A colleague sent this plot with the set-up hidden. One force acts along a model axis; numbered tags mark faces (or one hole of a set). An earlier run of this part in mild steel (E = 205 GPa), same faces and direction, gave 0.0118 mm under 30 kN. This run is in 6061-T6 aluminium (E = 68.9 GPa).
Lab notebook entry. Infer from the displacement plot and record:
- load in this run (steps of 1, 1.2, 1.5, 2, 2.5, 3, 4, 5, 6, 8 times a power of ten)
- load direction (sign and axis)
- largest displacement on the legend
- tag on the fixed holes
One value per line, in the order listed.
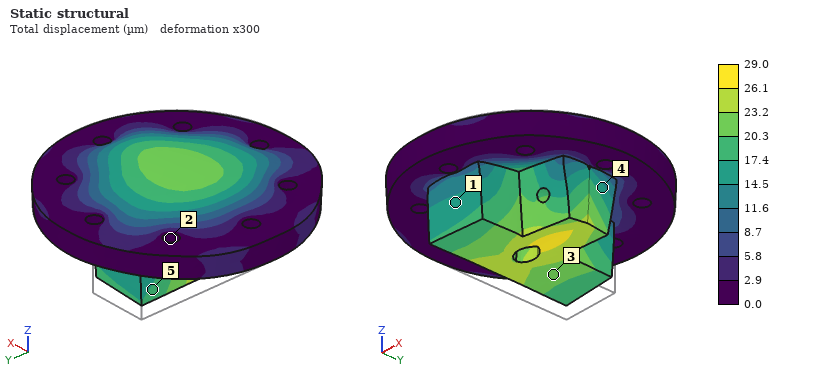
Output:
25 kN
+Z
29.0 µm
2
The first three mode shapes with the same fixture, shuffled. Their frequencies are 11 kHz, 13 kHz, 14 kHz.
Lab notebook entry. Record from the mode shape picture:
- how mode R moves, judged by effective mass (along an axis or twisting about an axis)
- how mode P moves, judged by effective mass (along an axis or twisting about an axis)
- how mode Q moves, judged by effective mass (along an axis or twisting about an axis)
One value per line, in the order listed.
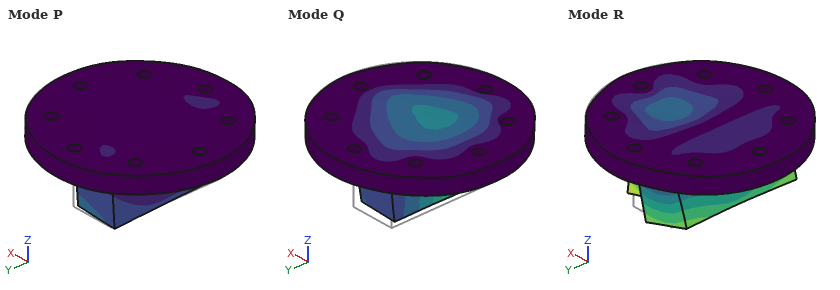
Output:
along X
along Y
along Z
